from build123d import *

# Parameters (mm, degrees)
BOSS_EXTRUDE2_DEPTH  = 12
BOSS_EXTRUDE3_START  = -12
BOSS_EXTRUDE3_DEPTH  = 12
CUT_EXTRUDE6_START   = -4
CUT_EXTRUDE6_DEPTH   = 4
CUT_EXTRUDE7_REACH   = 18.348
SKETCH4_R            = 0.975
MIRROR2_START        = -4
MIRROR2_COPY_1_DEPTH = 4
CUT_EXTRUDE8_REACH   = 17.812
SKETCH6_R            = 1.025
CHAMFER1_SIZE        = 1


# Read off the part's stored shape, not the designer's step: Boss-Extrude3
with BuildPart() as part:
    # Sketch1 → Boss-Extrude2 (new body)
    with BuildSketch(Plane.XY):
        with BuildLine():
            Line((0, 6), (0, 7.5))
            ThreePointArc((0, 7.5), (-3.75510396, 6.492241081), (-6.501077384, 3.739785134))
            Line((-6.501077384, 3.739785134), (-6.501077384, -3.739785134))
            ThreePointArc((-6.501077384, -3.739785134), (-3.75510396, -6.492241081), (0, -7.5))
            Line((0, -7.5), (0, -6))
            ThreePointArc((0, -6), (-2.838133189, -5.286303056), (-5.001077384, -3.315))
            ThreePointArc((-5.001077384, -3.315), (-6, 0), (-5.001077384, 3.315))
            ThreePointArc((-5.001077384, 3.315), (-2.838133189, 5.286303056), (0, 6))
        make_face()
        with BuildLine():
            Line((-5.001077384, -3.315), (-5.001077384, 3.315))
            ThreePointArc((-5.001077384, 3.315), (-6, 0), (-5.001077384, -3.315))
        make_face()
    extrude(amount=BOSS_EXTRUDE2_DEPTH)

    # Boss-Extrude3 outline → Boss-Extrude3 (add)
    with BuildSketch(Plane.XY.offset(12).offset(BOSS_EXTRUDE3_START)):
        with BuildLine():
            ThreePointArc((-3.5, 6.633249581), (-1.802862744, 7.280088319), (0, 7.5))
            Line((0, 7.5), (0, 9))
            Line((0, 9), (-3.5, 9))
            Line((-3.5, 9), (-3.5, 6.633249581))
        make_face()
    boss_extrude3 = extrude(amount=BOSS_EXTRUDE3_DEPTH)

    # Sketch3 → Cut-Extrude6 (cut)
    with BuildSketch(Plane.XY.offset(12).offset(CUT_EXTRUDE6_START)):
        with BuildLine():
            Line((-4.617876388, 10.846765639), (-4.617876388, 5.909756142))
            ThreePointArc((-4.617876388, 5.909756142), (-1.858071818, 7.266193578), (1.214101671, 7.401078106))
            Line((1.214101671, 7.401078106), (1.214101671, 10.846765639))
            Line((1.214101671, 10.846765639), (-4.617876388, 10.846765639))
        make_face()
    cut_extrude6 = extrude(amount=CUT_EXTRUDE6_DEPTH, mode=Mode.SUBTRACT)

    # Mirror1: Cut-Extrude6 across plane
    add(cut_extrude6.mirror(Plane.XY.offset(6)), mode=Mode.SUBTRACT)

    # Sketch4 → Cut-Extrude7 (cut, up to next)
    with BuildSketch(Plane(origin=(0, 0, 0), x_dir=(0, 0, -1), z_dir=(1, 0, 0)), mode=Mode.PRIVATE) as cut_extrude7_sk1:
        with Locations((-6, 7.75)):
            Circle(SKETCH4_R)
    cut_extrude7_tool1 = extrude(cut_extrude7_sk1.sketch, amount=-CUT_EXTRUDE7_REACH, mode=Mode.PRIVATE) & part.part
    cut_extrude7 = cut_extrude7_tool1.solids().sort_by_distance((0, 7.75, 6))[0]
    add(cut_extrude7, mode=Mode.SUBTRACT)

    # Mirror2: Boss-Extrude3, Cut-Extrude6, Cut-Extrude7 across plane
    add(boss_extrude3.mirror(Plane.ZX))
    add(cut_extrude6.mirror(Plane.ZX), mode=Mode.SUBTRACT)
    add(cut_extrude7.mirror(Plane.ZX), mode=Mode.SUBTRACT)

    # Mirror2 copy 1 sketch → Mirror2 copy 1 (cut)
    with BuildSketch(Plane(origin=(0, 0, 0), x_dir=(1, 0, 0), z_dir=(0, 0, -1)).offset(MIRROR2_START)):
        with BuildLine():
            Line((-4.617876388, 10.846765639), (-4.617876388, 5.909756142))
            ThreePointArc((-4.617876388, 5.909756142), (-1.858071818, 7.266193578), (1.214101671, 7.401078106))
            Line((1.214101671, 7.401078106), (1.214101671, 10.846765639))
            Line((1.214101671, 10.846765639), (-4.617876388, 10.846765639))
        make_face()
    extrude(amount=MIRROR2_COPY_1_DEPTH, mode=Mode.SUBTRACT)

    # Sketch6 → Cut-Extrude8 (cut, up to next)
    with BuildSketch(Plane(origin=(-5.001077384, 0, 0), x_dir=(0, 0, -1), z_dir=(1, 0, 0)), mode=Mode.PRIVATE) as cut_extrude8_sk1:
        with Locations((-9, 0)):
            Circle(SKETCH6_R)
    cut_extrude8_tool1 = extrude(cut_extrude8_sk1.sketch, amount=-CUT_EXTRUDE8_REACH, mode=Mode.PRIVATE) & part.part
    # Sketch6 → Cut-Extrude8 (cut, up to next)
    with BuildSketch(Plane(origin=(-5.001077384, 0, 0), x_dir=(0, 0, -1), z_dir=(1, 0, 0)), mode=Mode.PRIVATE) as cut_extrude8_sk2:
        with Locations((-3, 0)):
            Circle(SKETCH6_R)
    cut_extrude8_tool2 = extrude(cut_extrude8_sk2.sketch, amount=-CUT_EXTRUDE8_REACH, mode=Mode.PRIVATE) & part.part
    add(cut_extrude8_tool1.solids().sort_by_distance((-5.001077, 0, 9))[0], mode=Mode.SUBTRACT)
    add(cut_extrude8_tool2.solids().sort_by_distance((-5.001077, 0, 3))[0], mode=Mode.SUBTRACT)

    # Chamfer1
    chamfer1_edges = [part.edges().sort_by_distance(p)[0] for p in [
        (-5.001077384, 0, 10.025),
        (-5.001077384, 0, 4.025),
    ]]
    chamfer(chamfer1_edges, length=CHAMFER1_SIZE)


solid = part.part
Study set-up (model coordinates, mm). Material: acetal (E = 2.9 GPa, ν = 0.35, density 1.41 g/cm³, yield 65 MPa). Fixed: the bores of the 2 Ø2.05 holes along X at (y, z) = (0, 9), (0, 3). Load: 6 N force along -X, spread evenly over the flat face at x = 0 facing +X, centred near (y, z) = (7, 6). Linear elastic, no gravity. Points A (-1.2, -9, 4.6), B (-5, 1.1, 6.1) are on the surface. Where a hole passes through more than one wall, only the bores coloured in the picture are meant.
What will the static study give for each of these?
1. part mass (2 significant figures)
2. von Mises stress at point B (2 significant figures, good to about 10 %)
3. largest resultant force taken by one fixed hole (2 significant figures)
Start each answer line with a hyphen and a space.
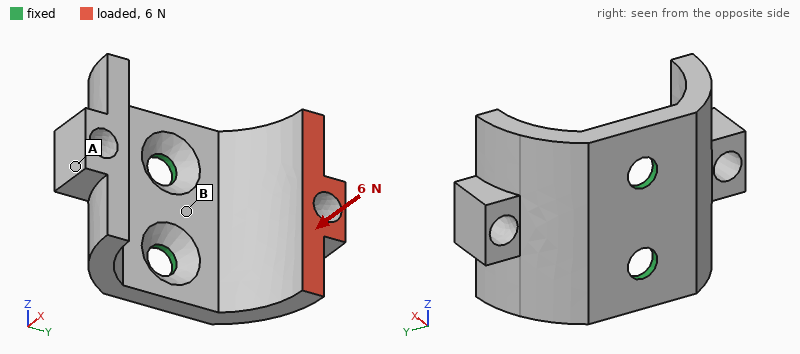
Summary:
- 0.54 g
- 9.5 MPa
- 3.0 N
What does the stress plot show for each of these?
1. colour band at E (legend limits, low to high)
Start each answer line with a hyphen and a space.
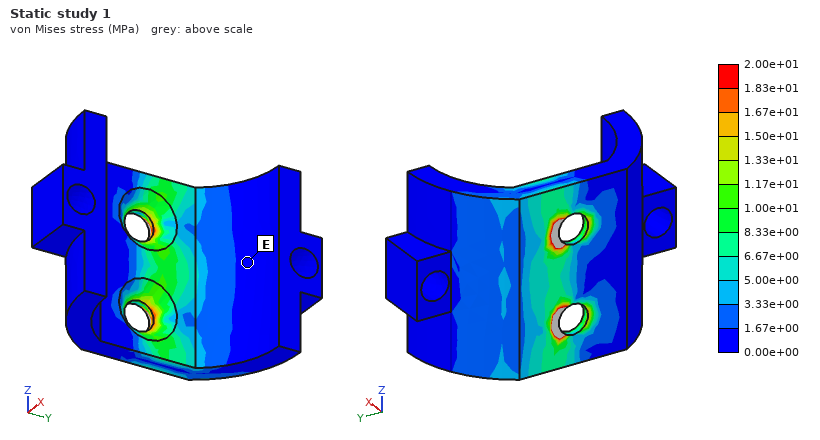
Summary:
- 0.00e+00 to 1.67e+00 MPa
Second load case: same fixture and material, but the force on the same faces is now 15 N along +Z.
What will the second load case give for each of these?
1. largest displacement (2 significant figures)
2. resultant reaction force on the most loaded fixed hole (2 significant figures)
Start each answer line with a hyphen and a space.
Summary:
- 0.14 mm
- 22 N
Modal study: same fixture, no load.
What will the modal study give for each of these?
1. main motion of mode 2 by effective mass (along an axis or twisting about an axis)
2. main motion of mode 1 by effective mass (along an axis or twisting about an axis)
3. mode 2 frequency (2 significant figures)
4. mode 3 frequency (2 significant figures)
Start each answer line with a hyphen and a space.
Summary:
- along X
- along Y
- 2900 Hz
- 5300 Hz
